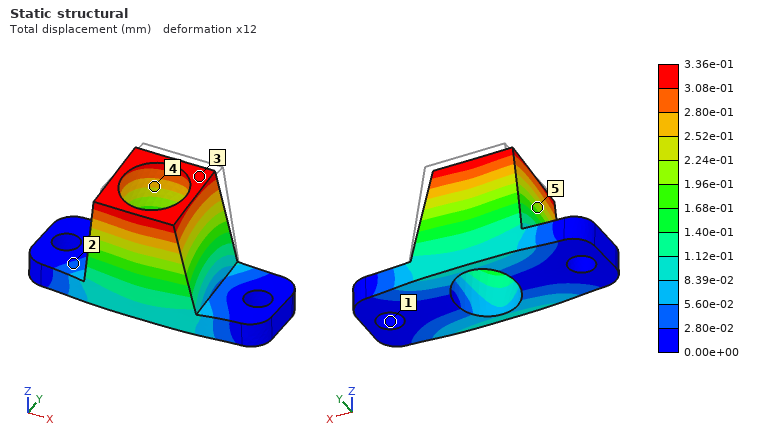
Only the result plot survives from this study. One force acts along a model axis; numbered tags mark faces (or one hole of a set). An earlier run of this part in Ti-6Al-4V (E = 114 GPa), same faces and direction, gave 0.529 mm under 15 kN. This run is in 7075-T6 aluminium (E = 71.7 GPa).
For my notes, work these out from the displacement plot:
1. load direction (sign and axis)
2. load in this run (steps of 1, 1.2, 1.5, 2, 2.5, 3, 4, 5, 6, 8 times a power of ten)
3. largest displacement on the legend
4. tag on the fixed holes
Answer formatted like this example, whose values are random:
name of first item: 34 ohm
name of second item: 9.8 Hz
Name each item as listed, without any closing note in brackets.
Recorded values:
load direction: -Y
load in this run: 6 kN
largest displacement on the legend: 3.36e-01 mm
tag on the fixed holes: 1
